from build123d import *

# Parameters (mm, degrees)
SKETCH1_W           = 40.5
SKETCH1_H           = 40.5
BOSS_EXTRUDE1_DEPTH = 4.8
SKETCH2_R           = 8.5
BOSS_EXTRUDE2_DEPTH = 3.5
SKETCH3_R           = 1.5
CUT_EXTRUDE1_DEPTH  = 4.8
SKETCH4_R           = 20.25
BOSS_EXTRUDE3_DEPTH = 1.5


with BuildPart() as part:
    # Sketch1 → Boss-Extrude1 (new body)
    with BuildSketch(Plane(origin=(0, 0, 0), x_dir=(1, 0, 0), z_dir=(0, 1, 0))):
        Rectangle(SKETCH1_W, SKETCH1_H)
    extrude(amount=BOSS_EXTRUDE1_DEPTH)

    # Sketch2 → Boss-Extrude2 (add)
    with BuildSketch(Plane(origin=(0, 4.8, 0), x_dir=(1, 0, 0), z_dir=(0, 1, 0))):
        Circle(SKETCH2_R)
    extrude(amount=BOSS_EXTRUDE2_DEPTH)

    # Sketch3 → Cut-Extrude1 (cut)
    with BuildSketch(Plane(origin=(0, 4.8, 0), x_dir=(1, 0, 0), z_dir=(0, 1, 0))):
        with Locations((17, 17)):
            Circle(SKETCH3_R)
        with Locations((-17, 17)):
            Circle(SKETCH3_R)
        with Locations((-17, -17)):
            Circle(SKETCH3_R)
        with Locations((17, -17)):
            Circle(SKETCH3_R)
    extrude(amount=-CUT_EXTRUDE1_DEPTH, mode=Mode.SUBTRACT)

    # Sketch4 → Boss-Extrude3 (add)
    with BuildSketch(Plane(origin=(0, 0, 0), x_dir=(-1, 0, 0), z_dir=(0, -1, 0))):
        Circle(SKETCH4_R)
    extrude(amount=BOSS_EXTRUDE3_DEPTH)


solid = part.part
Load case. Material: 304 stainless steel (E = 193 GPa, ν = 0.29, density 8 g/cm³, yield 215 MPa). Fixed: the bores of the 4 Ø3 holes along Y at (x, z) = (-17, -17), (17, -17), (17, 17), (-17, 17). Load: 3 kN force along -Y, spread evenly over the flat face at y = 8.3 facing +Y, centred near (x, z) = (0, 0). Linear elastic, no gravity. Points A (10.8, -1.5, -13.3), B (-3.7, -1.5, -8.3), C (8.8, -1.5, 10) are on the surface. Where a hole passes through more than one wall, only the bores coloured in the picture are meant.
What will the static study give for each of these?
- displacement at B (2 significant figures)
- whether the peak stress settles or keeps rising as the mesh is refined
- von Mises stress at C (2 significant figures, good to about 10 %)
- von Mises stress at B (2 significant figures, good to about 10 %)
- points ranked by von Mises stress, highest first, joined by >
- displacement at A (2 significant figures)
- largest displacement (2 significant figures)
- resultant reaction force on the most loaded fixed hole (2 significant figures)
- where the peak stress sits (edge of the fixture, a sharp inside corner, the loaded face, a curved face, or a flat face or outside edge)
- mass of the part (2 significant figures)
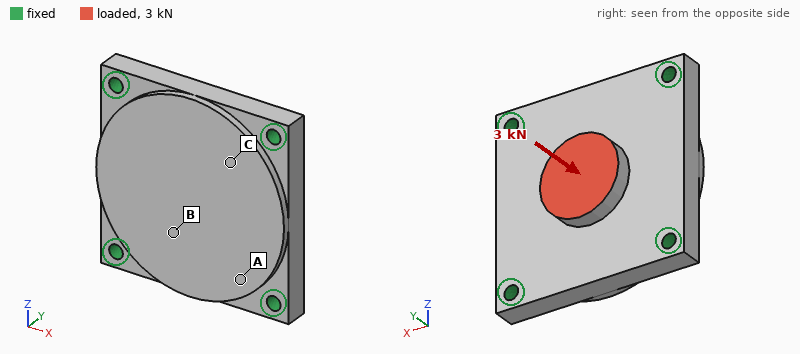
9.2 µm
keeps rising
23 MPa
40 MPa
B > C > A
4.8 µm
11 µm
790 N
edge of the fixture
84 g
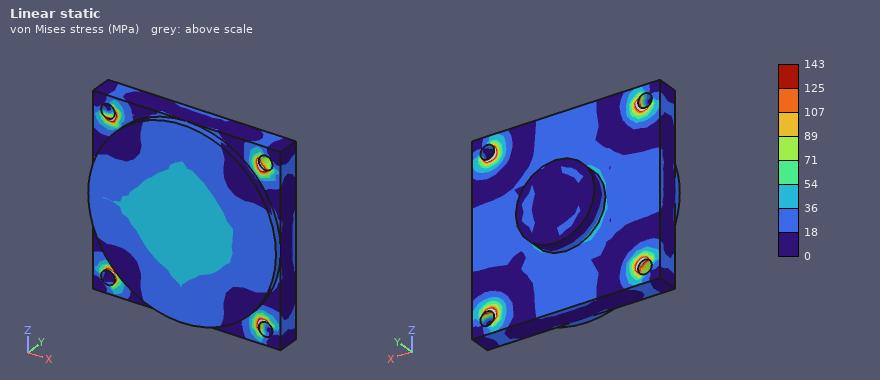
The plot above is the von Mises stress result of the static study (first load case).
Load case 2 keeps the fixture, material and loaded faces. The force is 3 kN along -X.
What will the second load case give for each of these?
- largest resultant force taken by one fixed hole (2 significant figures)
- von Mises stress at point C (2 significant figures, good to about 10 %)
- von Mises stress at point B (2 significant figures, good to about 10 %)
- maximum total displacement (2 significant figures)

850 N
10.0 MPa
11 MPa
6.0 µm
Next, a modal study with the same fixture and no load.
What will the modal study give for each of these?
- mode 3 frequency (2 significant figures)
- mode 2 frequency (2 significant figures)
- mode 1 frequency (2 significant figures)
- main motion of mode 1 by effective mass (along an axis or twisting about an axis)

22 kHz
22 kHz
13 kHz
along Y
